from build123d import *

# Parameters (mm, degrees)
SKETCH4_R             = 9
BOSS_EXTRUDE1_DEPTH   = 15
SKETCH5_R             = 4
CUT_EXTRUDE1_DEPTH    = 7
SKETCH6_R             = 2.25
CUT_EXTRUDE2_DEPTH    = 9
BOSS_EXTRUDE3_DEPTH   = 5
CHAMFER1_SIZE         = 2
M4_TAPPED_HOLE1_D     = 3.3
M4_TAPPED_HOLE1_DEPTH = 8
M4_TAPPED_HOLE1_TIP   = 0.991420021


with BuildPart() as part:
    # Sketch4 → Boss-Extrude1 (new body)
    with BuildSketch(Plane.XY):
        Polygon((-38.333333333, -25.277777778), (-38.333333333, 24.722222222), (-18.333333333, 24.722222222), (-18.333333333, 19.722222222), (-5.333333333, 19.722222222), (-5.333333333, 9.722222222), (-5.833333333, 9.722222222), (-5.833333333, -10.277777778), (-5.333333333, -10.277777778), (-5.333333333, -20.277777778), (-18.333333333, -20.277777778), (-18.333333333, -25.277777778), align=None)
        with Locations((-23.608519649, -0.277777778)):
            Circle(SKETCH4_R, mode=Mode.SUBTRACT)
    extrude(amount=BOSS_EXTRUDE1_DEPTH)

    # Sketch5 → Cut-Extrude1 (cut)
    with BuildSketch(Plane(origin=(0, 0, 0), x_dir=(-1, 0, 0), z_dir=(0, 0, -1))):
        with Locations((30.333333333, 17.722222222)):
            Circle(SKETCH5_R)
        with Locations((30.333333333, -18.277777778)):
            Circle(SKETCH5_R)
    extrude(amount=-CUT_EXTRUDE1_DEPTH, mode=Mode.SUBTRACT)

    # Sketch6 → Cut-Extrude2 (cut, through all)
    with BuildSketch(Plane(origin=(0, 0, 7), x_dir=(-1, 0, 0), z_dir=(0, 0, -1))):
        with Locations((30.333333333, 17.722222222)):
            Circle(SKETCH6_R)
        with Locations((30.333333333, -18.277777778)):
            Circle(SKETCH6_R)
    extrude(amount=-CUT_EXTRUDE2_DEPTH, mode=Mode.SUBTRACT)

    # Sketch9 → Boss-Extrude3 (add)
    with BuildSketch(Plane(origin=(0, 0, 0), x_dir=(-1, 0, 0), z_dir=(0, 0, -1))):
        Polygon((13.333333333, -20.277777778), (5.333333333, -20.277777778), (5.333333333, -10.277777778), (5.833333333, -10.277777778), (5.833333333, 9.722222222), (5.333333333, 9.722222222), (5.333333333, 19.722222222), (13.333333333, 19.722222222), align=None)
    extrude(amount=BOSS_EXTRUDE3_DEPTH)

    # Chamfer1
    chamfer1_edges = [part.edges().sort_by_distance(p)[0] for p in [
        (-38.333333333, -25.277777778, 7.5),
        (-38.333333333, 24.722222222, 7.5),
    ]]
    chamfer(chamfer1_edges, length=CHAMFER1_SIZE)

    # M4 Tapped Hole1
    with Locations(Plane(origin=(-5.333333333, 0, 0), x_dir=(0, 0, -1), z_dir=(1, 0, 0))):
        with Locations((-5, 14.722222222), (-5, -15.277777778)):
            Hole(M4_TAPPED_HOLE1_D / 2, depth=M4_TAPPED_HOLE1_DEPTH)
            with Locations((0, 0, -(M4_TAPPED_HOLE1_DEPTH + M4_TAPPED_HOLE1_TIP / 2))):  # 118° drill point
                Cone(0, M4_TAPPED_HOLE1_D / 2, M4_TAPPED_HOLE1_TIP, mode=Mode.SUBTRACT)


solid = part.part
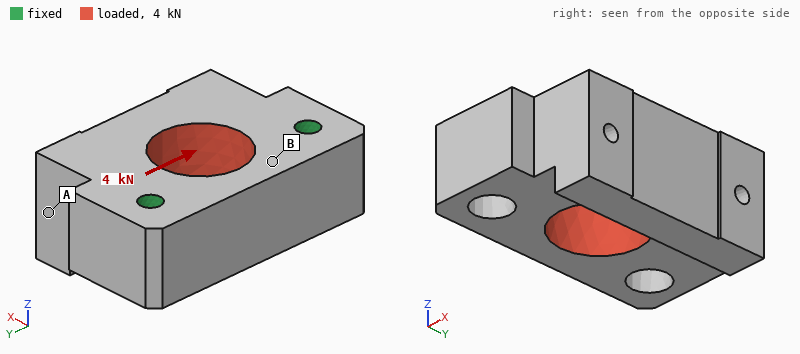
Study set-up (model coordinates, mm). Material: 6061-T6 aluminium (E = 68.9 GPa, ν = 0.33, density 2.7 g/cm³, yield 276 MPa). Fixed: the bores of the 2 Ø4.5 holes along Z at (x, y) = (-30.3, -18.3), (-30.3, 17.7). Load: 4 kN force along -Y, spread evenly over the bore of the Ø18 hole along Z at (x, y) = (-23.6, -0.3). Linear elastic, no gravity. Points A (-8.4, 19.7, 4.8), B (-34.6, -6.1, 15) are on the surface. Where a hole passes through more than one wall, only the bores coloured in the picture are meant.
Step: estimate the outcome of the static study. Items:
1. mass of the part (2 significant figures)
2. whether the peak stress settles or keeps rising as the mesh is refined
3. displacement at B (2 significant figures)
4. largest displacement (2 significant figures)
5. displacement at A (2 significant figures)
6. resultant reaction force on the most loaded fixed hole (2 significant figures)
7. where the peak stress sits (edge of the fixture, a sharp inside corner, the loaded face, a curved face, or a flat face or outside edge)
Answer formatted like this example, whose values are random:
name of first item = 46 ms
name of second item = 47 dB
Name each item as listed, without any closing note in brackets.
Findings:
mass of the part = 52 g
whether the peak stress settles or keeps rising as the mesh is refined = keeps rising
displacement at B = 1.5 µm
largest displacement = 7.8 µm
displacement at A = 7.1 µm
resultant reaction force on the most loaded fixed hole = 2.1 kN
where the peak stress sits = edge of the fixture
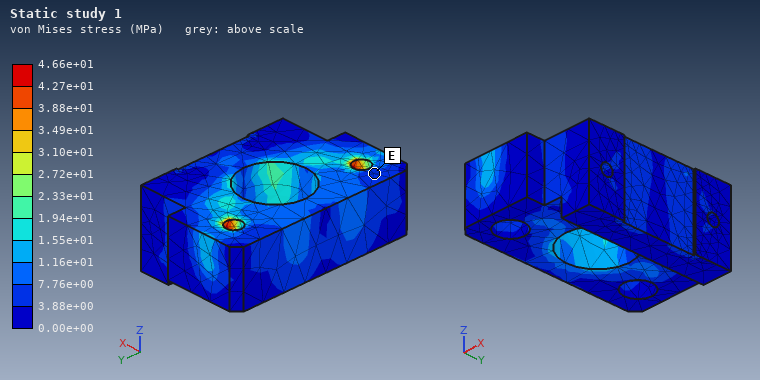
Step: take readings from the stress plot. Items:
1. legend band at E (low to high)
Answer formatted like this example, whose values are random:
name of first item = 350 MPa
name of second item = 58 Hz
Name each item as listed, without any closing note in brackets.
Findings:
legend band at E = 3.88e+00 to 7.76e+00 MPa
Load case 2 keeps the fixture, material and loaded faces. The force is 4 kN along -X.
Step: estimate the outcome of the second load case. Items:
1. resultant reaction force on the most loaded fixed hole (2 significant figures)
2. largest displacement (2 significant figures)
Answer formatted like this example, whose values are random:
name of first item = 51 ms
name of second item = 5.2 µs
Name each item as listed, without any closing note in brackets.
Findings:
resultant reaction force on the most loaded fixed hole = 2.0 kN
largest displacement = 17 µm
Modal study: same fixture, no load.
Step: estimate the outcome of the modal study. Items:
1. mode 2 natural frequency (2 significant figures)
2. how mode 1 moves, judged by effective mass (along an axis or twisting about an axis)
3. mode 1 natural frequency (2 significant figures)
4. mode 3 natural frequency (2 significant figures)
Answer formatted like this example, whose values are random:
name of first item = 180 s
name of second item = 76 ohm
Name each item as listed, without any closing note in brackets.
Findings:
mode 2 natural frequency = 16 kHz
how mode 1 moves, judged by effective mass = along Z
mode 1 natural frequency = 7200 Hz
mode 3 natural frequency = 16 kHz
